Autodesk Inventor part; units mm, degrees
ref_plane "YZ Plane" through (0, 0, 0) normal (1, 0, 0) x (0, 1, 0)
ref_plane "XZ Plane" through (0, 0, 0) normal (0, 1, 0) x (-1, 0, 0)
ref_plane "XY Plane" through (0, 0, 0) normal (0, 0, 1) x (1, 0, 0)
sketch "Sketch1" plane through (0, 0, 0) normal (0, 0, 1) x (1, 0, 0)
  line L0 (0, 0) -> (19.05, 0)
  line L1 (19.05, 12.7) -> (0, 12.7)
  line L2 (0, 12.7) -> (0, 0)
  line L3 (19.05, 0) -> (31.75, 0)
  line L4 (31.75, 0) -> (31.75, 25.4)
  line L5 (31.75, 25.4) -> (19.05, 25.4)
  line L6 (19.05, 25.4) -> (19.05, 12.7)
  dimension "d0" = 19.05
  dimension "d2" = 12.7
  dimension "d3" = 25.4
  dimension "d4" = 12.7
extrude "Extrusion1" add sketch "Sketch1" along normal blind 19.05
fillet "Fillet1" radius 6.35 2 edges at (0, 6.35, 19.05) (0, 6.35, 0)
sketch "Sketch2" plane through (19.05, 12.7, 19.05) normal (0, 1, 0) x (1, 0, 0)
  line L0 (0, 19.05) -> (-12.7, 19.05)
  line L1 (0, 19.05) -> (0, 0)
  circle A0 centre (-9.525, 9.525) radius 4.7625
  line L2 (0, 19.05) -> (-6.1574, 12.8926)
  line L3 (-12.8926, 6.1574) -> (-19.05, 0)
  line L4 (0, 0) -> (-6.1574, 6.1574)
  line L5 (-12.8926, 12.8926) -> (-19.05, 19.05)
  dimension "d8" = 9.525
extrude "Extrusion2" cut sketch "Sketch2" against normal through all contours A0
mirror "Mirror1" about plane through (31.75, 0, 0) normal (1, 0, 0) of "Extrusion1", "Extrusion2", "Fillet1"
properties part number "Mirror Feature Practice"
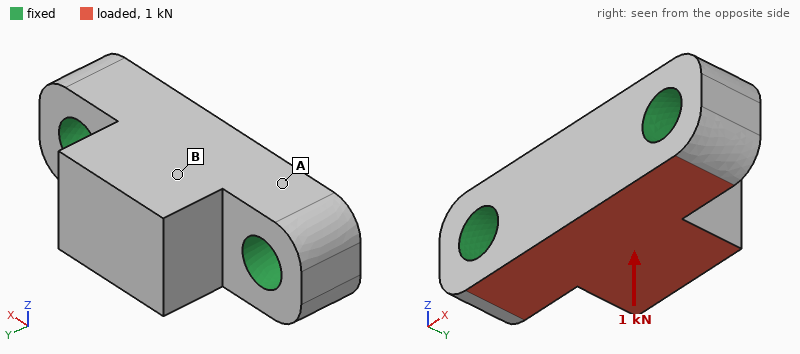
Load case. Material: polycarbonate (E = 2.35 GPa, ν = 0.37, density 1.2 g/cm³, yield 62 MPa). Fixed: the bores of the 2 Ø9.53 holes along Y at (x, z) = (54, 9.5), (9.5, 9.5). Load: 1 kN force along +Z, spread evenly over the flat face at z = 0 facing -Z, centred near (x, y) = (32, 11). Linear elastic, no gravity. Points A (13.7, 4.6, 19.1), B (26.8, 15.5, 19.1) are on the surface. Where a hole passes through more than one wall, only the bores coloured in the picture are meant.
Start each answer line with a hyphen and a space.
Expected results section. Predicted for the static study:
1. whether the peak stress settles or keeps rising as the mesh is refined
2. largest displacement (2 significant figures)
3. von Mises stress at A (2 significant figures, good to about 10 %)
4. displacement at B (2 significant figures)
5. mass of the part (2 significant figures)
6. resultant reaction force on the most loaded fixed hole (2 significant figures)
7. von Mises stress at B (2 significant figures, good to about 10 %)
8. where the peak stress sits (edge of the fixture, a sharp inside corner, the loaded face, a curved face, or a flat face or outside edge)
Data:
- keeps rising
- 0.11 mm
- 3.4 MPa
- 0.068 mm
- 23 g
- 500 N
- 1.4 MPa
- edge of the fixture
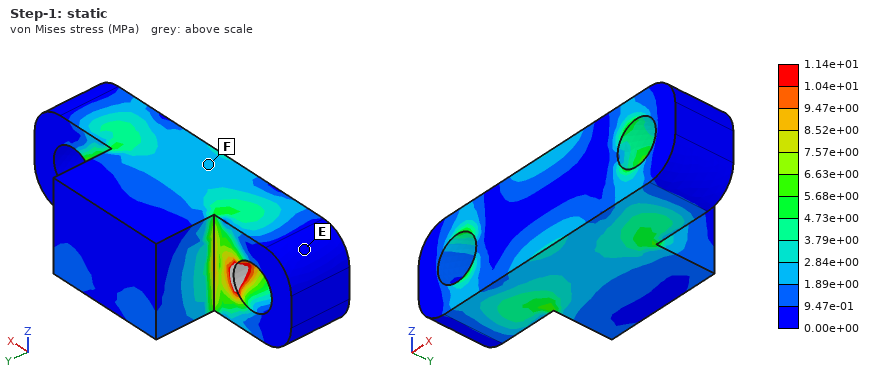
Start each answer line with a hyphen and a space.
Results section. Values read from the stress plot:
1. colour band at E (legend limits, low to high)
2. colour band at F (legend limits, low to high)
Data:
- 0.00e+00 to 9.47e-01 MPa
- 1.89e+00 to 2.84e+00 MPa
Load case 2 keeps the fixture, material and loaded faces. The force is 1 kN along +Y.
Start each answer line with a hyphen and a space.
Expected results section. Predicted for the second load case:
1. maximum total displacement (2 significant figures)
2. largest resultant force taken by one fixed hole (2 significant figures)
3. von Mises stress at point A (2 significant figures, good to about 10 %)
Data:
- 0.14 mm
- 510 N
- 3.2 MPa
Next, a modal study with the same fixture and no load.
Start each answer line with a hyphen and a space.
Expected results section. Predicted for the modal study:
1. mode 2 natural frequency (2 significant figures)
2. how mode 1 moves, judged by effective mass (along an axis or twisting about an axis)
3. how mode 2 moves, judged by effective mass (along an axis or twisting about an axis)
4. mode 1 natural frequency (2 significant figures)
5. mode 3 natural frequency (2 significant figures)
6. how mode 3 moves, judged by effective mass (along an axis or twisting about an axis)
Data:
- 6700 Hz
- along Z
- along Y
- 3900 Hz
- 8100 Hz
- along X
